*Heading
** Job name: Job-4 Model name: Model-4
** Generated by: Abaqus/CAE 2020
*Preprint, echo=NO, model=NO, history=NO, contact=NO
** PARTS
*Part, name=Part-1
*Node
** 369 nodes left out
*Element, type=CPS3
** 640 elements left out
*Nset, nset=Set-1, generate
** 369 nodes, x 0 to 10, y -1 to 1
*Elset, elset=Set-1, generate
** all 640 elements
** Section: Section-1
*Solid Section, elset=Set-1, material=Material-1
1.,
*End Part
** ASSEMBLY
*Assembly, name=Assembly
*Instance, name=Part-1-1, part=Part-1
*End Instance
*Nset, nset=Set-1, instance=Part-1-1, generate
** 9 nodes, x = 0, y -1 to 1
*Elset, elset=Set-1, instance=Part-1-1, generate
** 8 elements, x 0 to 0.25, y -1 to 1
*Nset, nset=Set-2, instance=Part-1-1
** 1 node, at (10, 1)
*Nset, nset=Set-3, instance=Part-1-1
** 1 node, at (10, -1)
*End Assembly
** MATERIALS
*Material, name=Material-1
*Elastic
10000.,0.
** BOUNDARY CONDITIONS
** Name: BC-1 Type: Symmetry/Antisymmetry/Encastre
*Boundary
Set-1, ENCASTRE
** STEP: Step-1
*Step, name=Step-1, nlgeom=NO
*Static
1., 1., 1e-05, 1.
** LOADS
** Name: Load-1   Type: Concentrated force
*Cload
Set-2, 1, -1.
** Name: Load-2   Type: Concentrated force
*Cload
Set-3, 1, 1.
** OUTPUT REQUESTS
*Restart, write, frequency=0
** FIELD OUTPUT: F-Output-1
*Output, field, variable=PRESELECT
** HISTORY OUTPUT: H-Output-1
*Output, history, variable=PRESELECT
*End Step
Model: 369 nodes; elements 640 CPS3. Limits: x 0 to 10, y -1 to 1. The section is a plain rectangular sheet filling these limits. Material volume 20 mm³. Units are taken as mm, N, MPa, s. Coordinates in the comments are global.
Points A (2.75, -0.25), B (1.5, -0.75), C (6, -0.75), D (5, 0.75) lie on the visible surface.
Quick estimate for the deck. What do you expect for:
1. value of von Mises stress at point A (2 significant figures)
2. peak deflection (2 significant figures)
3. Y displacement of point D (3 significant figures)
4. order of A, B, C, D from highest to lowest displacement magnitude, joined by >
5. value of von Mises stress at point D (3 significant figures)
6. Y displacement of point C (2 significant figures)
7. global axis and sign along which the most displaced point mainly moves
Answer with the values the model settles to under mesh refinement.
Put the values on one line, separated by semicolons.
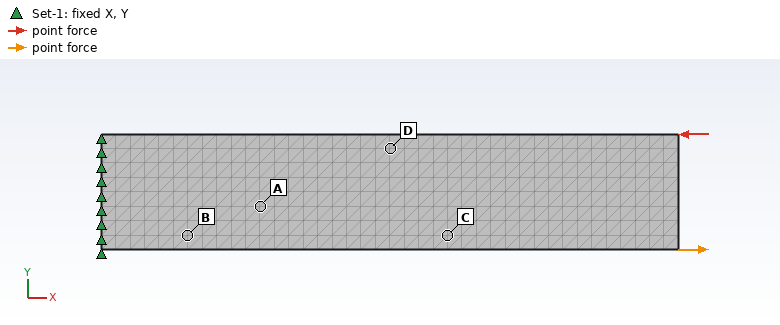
0.75 MPa; 0.016 mm; 0.00375 mm; C > D > A > B; 2.25 MPa; 0.0054 mm; +Y
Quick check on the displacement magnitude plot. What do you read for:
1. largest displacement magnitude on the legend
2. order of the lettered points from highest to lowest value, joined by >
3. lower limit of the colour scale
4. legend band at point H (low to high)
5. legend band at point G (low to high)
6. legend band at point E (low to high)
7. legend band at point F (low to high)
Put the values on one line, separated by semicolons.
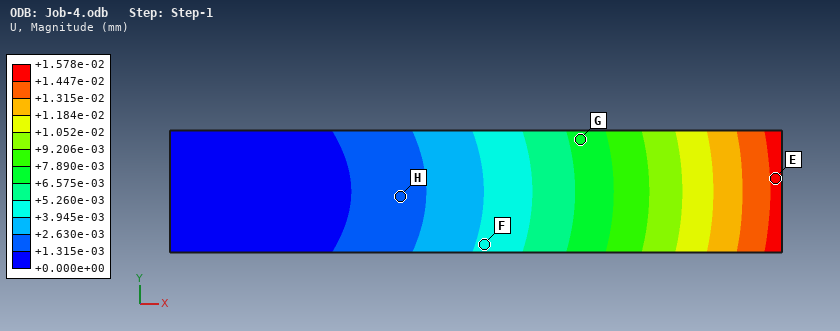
+1.578e-02 mm; E > G > F > H; +0.000e+00 mm; +1.315e-03 to +2.630e-03 mm; +6.575e-03 to +7.890e-03 mm; +1.447e-02 to +1.578e-02 mm; +3.945e-03 to +5.260e-03 mm
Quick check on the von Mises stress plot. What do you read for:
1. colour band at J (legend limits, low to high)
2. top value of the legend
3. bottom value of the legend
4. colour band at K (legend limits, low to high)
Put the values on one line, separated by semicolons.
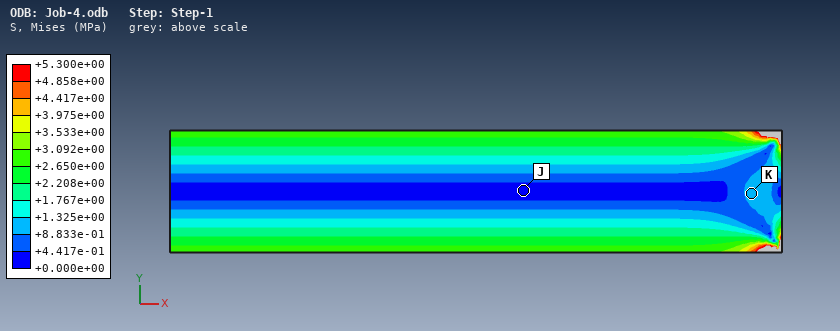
+0.000e+00 to +4.417e-01 MPa; +5.300e+00 MPa; +0.000e+00 MPa; +8.833e-01 to +1.325e+00 MPa
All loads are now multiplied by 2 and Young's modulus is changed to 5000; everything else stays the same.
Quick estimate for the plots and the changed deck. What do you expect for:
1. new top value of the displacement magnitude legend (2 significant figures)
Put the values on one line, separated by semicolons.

0.063 mm
